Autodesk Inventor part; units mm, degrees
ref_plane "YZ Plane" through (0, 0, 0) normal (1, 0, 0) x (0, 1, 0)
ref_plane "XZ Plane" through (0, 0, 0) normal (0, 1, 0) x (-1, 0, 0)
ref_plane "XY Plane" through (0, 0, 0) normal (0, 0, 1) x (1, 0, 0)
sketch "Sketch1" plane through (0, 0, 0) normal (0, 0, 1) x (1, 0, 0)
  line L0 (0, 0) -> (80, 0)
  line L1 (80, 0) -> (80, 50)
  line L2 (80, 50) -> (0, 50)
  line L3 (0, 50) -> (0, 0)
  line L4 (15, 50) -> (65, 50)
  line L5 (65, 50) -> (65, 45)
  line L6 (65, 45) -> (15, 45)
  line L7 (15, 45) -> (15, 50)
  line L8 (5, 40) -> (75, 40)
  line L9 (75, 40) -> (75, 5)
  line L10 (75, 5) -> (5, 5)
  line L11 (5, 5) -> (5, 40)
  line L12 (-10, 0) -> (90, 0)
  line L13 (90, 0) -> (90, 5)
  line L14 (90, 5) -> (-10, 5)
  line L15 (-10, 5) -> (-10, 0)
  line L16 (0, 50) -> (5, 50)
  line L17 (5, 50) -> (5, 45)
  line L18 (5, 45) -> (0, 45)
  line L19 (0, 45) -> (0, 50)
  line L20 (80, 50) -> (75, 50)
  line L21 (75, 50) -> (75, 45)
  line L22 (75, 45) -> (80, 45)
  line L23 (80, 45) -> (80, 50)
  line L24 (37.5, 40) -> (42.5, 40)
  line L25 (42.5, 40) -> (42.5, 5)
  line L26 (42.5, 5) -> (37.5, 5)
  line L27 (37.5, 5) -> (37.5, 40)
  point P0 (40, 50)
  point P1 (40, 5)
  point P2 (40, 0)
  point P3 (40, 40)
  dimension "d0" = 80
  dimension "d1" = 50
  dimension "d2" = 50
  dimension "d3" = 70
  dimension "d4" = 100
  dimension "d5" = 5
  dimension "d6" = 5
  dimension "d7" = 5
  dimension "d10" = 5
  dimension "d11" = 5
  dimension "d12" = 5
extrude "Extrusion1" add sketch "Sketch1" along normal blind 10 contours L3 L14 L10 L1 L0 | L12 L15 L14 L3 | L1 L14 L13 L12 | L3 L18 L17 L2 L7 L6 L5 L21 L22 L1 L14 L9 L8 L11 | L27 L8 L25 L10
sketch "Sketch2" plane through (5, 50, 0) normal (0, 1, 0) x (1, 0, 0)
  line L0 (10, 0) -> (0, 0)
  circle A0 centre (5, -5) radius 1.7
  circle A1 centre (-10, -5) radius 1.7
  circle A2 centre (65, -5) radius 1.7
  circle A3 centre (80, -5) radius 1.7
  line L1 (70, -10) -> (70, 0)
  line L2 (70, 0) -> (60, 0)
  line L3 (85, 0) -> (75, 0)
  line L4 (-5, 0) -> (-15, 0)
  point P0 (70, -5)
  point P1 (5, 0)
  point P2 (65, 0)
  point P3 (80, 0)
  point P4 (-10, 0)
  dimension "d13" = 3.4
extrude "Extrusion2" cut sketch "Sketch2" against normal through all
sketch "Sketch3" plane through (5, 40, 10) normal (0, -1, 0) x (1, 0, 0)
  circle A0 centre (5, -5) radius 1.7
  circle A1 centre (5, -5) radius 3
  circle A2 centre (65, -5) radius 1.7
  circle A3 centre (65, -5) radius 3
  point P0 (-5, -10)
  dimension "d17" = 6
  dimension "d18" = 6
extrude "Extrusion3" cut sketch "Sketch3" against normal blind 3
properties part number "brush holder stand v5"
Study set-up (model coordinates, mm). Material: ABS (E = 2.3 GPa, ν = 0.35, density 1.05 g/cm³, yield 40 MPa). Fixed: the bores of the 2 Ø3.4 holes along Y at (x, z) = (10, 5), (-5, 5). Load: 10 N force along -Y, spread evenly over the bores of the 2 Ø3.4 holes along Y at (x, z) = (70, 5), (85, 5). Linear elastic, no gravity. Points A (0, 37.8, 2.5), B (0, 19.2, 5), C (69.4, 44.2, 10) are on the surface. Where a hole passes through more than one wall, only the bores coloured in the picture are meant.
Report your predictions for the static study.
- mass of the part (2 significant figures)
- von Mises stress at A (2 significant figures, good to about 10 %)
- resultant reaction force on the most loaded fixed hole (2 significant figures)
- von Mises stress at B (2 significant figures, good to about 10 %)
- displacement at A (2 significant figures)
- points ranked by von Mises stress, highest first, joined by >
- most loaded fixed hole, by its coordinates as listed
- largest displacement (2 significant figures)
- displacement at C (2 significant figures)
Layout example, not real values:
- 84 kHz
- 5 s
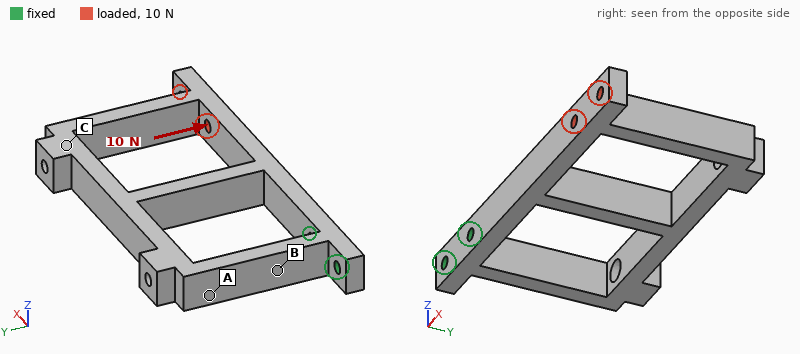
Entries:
- 16 g
- 1.5 MPa
- 40 N
- 2.8 MPa
- 0.40 mm
- B > A > C
- (10, 5)
- 1.1 mm
- 0.98 mm
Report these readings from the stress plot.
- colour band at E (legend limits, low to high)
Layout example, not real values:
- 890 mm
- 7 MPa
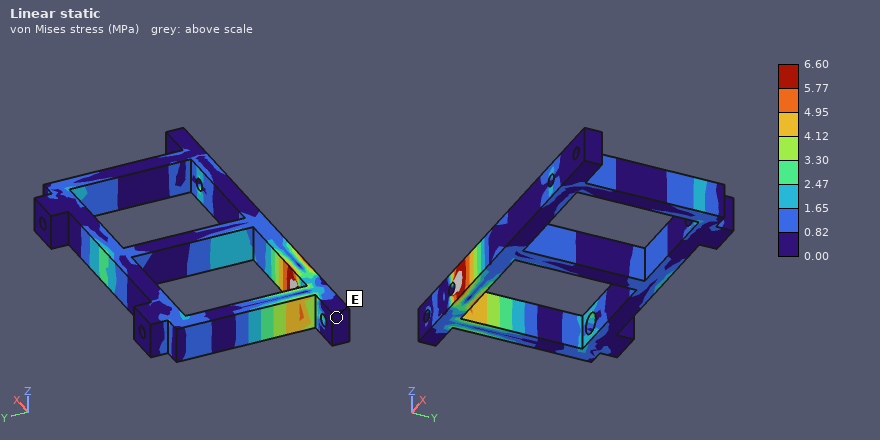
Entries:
- 0.00 to 0.82 MPa
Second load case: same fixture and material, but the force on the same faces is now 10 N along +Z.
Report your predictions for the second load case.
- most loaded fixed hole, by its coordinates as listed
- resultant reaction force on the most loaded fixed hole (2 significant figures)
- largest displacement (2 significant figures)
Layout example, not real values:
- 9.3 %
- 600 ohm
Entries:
- (10, 5)
- 33 N
- 1.2 mm
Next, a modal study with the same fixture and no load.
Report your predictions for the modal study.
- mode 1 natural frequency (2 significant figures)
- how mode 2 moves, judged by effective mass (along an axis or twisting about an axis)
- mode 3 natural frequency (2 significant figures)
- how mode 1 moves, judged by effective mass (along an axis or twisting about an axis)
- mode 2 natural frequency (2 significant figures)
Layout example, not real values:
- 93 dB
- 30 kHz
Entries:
- 180 Hz
- along Y
- 420 Hz
- along Z
- 190 Hz
